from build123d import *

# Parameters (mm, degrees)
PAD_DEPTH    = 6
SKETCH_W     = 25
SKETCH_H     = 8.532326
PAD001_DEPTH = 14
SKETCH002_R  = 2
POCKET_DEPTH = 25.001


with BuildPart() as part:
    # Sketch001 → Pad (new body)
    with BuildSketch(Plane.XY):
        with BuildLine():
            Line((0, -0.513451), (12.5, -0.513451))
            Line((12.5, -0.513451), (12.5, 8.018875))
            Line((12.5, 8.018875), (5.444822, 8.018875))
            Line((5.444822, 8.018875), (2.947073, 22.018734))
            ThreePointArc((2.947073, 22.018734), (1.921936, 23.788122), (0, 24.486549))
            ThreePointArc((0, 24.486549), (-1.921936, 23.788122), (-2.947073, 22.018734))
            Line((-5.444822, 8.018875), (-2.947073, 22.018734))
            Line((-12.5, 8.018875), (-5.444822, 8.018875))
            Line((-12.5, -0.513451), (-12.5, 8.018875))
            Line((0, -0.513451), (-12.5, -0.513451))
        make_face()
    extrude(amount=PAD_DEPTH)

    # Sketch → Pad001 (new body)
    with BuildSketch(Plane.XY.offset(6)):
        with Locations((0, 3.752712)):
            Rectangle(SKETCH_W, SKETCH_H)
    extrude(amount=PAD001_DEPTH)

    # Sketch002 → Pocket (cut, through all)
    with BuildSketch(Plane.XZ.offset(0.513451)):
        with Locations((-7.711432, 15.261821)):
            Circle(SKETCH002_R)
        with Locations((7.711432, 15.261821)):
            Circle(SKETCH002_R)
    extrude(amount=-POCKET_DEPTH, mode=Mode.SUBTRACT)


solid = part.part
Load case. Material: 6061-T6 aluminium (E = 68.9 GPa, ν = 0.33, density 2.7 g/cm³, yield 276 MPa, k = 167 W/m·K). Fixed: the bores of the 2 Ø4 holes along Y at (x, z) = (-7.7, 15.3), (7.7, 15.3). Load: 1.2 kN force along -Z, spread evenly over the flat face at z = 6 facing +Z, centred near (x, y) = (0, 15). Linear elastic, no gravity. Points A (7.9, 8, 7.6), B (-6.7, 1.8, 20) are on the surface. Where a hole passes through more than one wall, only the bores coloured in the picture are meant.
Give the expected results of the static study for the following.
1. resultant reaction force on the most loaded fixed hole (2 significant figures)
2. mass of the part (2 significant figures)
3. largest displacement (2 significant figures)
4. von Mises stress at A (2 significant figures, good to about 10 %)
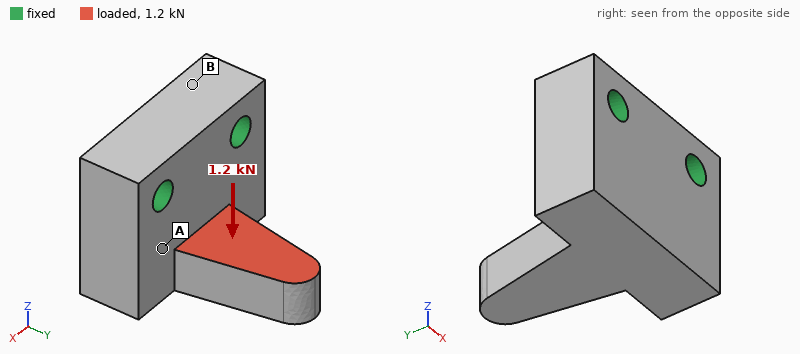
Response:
660 N
13 g
0.12 mm
44 MPa
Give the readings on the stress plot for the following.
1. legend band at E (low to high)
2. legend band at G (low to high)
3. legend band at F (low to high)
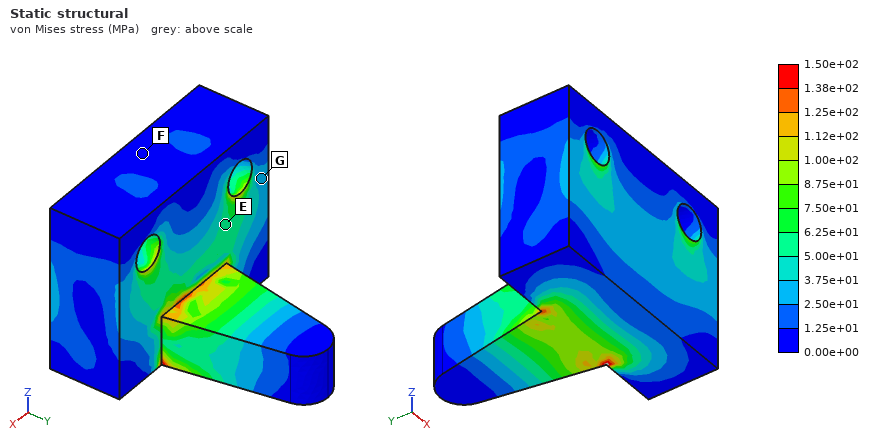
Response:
5.00e+01 to 6.25e+01 MPa
2.50e+01 to 3.75e+01 MPa
0.00e+00 to 1.25e+01 MPa
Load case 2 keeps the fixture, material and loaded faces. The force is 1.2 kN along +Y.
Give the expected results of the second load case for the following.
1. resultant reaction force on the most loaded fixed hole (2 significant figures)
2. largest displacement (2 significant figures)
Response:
600 N
27 µm
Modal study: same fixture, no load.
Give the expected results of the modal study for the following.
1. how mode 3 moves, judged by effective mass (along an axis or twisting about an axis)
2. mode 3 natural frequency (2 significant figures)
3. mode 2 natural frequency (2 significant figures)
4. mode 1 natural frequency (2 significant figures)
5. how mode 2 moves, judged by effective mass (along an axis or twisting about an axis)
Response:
along Y
24 kHz
19 kHz
13 kHz
along X
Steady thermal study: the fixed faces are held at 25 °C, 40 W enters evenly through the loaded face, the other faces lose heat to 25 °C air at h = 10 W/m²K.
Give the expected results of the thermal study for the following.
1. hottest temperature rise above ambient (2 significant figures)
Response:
56 K
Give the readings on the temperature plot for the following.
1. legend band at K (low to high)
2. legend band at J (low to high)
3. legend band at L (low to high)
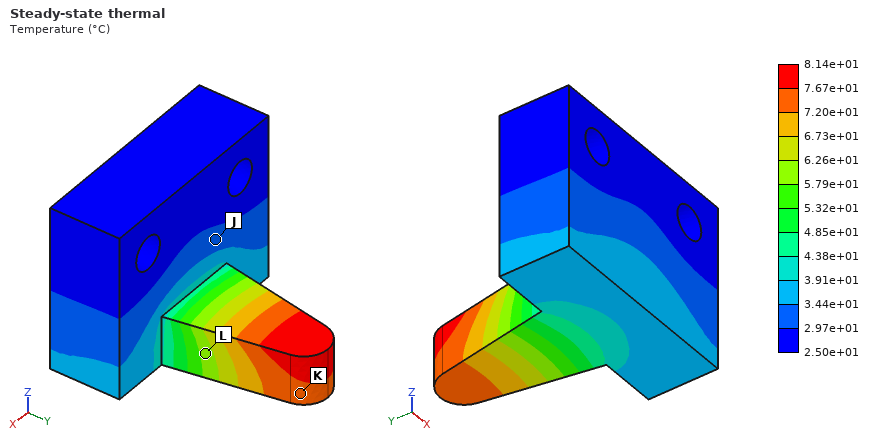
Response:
7.20e+01 to 7.67e+01 °C
2.97e+01 to 3.44e+01 °C
5.79e+01 to 6.26e+01 °C
